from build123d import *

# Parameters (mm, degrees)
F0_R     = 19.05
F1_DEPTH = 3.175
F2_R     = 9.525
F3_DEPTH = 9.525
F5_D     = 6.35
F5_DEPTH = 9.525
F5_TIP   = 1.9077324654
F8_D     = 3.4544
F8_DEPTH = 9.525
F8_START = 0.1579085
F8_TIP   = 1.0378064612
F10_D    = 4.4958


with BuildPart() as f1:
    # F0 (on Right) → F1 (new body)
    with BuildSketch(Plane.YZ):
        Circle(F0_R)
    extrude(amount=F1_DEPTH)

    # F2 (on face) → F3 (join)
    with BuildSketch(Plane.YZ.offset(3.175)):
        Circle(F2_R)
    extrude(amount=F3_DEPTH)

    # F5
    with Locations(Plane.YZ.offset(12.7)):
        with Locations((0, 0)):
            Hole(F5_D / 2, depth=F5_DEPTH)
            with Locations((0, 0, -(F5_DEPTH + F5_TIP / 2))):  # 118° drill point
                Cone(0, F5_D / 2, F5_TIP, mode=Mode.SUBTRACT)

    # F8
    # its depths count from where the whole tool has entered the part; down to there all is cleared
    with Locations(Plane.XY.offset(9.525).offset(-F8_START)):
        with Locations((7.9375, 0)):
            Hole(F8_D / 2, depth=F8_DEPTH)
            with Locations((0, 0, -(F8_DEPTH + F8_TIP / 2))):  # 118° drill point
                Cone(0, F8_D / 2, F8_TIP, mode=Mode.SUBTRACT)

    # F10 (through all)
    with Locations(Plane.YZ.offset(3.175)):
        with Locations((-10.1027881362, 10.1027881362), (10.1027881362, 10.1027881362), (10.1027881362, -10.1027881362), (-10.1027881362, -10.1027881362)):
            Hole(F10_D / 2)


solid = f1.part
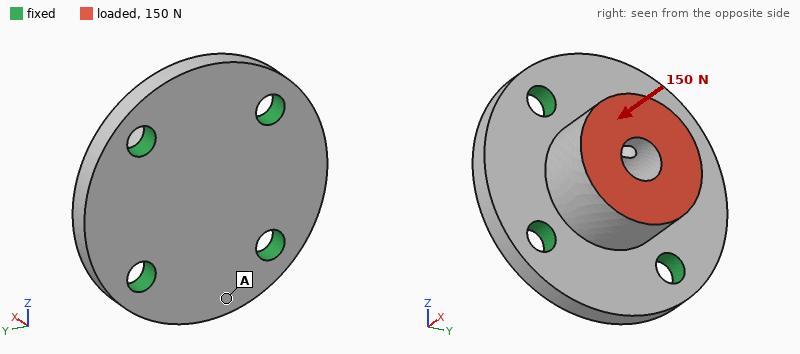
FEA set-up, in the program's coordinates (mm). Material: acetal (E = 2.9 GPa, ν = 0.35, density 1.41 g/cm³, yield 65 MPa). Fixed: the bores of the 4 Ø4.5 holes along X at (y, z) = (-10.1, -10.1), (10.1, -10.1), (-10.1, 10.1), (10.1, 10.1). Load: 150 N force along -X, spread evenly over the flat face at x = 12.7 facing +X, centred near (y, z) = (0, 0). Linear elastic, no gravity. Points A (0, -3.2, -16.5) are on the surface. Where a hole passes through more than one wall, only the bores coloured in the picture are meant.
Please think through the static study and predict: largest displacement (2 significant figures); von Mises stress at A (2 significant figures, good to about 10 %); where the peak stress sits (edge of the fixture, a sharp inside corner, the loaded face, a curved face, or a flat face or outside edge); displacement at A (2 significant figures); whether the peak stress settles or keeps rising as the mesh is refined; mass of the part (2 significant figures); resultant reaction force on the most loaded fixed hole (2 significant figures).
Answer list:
13 µm
0.56 MPa
edge of the fixture
2.6 µm
keeps rising
8.1 g
40 N
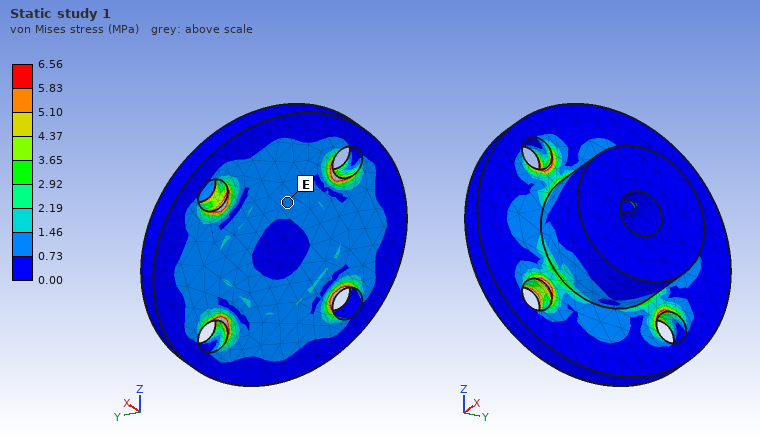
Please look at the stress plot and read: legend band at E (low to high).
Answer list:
0.73 to 1.46 MPa
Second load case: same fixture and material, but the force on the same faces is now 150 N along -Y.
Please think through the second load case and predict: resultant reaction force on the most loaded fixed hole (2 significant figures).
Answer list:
63 N
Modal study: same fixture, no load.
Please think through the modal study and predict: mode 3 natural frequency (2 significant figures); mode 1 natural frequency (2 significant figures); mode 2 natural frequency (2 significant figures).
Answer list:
8200 Hz
7900 Hz
8000 Hz
